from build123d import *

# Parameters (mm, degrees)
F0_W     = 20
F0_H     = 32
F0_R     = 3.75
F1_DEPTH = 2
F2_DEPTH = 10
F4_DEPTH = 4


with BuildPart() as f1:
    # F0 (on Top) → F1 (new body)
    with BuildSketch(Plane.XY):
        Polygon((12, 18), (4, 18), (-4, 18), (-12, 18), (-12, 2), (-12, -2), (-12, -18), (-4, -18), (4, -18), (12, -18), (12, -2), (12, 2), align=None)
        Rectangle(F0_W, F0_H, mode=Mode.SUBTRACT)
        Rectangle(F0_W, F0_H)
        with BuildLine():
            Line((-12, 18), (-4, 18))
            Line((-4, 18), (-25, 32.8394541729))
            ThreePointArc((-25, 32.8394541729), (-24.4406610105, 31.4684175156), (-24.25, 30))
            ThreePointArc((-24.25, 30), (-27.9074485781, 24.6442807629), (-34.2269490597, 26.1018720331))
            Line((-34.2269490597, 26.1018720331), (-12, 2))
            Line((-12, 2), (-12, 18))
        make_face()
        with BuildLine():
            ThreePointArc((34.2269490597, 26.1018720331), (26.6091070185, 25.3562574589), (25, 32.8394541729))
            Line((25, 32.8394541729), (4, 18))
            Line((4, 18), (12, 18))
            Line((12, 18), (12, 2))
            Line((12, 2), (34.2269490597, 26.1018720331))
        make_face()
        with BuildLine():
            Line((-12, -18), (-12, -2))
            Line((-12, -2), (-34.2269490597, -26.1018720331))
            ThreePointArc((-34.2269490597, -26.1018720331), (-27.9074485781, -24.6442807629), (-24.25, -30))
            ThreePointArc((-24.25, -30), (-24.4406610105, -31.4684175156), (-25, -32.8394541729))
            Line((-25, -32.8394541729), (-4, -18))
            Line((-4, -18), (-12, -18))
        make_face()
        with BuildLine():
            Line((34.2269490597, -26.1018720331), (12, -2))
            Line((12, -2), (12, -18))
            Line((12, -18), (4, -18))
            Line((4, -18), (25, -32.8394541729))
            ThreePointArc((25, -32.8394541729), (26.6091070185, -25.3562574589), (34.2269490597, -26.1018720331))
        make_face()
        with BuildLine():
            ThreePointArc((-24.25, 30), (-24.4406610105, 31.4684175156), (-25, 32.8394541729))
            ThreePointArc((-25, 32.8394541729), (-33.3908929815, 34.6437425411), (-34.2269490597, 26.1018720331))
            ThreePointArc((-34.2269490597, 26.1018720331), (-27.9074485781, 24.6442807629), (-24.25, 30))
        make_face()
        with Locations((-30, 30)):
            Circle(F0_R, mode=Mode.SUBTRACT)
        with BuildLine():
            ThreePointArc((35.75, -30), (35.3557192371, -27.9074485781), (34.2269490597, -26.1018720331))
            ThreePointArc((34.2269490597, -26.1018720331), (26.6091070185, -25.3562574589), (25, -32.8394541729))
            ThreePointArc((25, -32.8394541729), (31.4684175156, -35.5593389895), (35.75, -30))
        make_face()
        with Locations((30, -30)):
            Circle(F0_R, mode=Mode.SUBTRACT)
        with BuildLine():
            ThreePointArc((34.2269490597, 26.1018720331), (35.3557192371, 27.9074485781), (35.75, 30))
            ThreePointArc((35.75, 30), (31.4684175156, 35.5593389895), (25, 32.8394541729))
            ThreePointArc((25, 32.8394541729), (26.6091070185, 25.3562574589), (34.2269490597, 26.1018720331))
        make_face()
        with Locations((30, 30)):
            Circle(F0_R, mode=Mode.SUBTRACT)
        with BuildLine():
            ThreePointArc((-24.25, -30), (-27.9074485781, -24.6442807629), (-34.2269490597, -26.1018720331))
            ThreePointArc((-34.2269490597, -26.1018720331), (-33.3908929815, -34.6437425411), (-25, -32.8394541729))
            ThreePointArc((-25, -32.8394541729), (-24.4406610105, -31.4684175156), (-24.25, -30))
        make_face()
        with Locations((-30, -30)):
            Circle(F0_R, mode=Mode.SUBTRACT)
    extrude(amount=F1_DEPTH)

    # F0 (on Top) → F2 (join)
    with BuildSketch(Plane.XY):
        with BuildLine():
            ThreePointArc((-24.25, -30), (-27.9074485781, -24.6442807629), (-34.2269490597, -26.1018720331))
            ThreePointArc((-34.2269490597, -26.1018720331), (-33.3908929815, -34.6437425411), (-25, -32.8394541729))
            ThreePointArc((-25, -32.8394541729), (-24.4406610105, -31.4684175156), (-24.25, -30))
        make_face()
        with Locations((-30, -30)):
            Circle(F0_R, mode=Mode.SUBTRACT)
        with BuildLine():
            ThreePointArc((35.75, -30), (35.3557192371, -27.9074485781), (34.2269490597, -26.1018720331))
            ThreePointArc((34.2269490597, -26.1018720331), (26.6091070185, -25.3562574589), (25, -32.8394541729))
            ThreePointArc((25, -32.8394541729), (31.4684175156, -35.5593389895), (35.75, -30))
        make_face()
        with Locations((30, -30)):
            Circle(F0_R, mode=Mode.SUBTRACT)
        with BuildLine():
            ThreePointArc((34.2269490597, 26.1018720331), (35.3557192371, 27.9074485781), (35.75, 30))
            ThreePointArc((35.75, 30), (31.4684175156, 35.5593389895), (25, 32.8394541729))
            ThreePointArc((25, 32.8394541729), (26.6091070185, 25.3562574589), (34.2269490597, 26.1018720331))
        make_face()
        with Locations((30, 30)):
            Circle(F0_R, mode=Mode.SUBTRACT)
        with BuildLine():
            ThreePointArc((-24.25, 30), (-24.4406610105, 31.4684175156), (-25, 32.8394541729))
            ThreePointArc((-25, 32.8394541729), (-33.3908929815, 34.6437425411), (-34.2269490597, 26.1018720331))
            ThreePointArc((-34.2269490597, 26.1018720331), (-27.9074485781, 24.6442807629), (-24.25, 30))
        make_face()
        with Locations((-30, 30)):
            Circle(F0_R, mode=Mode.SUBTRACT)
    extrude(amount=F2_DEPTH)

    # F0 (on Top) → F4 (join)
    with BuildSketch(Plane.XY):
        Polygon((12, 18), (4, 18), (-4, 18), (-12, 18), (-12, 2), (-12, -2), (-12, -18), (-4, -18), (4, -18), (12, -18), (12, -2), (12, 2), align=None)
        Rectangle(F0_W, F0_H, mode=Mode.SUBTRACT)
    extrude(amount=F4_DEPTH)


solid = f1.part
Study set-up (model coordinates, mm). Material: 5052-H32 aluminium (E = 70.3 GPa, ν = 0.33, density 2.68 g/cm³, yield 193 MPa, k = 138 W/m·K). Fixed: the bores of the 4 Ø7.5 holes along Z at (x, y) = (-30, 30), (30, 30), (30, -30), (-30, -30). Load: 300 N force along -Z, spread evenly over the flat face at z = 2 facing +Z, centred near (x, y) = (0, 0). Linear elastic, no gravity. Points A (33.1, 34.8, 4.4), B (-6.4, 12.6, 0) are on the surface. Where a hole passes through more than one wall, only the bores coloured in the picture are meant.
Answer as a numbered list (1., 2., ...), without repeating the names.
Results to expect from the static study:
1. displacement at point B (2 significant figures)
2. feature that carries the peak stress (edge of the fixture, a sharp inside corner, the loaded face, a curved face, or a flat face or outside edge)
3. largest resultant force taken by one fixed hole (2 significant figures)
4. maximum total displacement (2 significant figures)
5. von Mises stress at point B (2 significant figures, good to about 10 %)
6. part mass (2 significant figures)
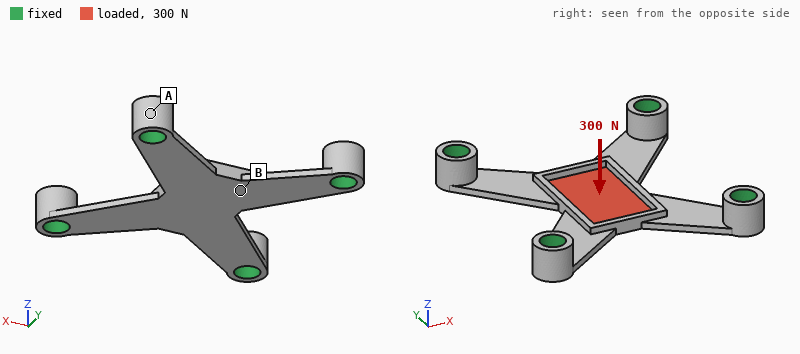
1. 0.16 mm
2. a flat face or outside edge
3. 100 N
4. 0.20 mm
5. 33 MPa
6. 19 g
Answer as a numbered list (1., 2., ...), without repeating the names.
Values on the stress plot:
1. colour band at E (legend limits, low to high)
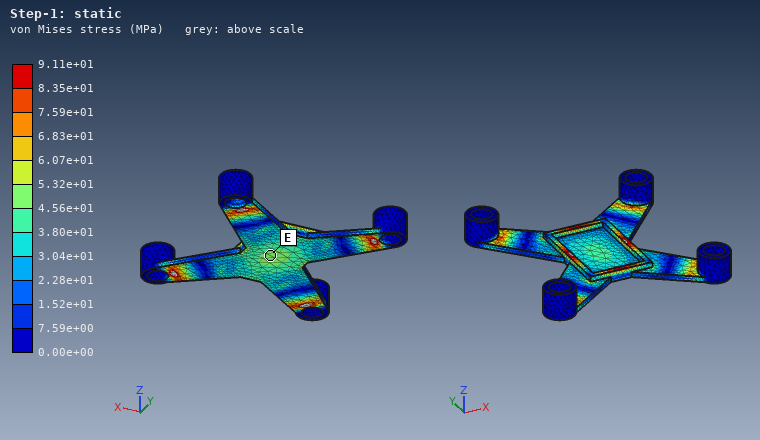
1. 4.56e+01 to 5.32e+01 MPa
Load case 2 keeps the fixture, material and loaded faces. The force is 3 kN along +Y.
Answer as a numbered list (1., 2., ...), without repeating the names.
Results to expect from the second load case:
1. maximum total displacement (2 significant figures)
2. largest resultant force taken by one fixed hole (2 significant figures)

1. 59 µm
2. 1.0 kN
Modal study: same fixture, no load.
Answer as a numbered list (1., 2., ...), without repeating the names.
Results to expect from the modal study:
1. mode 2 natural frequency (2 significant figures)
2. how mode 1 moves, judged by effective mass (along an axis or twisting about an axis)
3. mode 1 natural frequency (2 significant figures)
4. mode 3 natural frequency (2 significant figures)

1. 5100 Hz
2. along Z
3. 2500 Hz
4. 5500 Hz
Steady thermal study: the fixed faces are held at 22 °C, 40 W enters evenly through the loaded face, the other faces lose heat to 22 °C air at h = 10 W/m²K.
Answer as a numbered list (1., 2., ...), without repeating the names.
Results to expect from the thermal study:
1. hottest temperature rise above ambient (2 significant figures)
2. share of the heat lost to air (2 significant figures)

1. 72 K
2. 4.8 %
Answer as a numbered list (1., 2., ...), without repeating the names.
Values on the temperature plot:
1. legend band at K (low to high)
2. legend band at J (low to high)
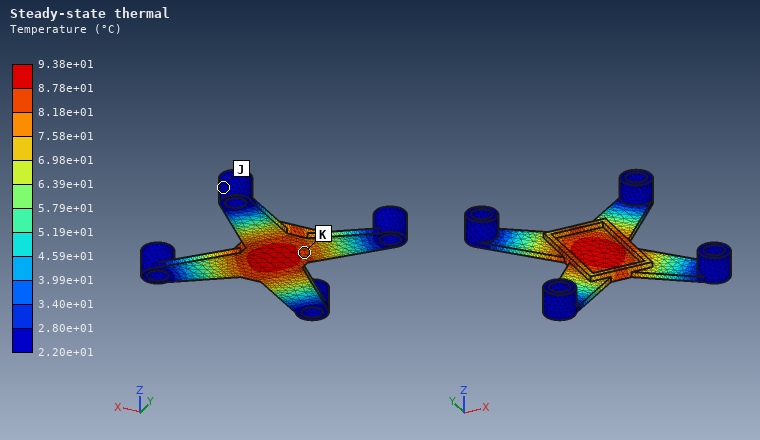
1. 8.18e+01 to 8.78e+01 °C
2. 2.20e+01 to 2.80e+01 °C
